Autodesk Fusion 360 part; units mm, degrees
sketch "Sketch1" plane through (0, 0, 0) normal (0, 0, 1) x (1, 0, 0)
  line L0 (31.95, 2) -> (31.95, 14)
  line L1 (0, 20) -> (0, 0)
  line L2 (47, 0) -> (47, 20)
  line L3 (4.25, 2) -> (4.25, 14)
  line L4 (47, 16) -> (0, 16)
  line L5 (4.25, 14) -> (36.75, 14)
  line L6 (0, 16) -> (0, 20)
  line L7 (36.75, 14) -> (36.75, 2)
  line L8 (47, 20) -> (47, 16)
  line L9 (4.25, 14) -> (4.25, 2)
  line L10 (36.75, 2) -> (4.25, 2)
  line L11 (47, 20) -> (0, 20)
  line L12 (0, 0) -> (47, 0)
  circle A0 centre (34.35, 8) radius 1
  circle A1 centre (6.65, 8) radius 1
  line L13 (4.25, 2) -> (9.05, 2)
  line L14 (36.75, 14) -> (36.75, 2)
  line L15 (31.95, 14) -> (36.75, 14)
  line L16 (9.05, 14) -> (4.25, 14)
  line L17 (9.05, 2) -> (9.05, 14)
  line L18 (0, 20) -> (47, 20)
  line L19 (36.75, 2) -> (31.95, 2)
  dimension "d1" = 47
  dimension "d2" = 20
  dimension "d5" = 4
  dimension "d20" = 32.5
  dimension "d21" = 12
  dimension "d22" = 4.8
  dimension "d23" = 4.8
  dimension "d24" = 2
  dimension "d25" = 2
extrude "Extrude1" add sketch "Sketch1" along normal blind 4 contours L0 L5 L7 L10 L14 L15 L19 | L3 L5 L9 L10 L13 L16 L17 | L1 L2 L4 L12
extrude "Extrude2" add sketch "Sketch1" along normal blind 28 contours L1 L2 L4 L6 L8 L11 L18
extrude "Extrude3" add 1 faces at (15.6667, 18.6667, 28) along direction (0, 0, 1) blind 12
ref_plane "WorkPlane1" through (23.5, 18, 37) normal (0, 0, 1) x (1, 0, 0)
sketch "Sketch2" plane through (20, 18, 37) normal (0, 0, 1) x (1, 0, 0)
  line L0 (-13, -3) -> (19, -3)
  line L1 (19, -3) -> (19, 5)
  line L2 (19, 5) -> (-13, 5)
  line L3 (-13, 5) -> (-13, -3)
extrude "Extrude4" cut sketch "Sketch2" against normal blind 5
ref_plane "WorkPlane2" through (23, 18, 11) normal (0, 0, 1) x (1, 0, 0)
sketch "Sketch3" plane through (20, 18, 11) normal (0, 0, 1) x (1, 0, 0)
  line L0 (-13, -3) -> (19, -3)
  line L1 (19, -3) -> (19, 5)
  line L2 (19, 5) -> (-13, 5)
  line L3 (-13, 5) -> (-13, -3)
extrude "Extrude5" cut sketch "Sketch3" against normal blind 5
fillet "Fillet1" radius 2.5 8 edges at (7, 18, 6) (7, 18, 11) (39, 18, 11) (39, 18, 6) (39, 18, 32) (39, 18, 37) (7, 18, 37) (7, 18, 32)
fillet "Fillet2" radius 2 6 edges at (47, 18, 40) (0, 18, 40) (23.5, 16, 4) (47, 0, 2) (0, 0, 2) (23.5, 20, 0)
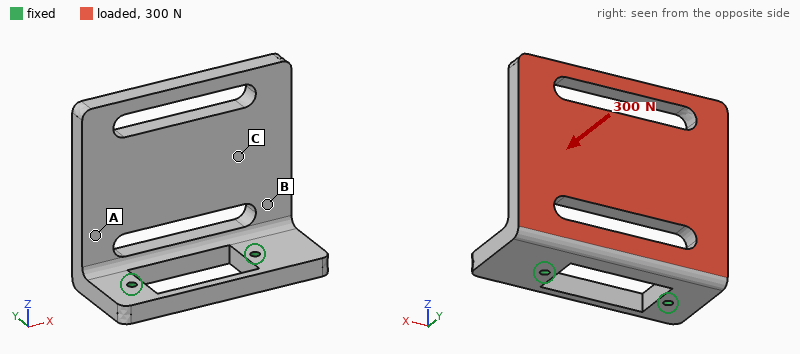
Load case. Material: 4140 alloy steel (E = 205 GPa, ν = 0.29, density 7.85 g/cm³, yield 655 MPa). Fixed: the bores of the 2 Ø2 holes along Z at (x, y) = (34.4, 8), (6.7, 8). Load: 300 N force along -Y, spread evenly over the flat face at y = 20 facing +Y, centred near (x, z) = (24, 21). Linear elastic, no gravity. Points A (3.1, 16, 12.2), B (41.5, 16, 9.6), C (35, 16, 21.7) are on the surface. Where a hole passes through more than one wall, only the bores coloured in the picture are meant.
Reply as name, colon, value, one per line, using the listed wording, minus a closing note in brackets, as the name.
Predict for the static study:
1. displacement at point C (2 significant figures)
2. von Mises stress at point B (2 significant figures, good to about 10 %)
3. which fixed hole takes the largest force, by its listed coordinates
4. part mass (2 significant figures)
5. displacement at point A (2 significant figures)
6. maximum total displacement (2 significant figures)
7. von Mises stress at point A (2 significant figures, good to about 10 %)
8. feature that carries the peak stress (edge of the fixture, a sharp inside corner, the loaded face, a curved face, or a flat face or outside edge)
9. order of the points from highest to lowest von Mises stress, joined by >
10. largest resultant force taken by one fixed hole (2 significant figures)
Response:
displacement at point C: 0.079 mm
von Mises stress at point B: 84 MPa
which fixed hole takes the largest force, by its listed coordinates: (34.4, 8)
part mass: 64 g
displacement at point A: 0.033 mm
maximum total displacement: 0.18 mm
von Mises stress at point A: 63 MPa
feature that carries the peak stress: a flat face or outside edge
order of the points from highest to lowest von Mises stress, joined by >: B > A > C
largest resultant force taken by one fixed hole: 170 N
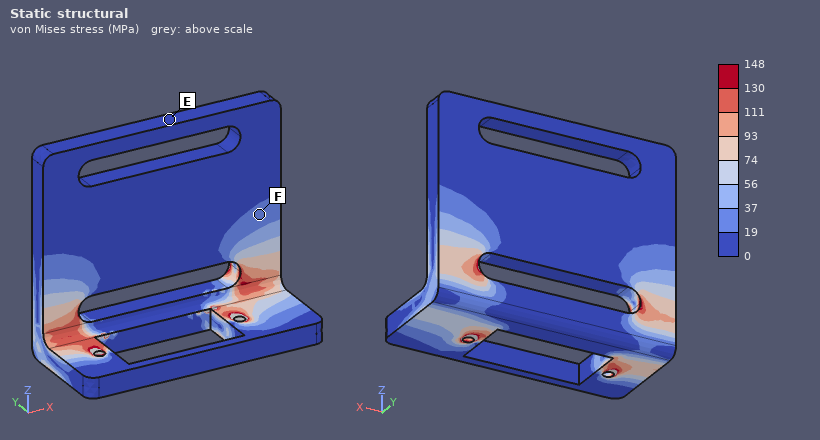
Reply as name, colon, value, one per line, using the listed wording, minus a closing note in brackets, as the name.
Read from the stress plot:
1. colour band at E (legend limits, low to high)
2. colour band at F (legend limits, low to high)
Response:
colour band at E: 0 to 19 MPa
colour band at F: 19 to 37 MPa
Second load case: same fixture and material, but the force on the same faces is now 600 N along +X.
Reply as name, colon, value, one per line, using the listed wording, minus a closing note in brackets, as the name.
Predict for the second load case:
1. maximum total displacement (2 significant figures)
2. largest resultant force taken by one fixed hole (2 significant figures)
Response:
maximum total displacement: 30 µm
largest resultant force taken by one fixed hole: 470 N
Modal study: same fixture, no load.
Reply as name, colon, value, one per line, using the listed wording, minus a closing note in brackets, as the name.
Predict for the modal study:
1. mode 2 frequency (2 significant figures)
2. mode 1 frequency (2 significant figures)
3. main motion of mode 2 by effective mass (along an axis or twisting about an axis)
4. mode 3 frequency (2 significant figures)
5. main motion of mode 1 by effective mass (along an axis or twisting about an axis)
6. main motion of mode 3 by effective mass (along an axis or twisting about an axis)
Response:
mode 2 frequency: 3300 Hz
mode 1 frequency: 1200 Hz
main motion of mode 2 by effective mass: along X
mode 3 frequency: 4300 Hz
main motion of mode 1 by effective mass: along Y
main motion of mode 3 by effective mass: along X
